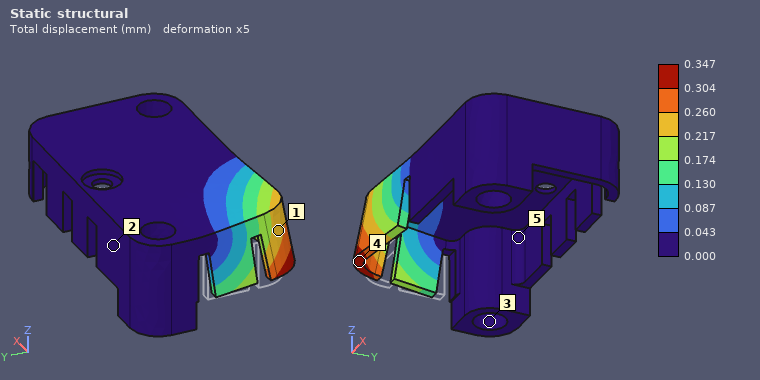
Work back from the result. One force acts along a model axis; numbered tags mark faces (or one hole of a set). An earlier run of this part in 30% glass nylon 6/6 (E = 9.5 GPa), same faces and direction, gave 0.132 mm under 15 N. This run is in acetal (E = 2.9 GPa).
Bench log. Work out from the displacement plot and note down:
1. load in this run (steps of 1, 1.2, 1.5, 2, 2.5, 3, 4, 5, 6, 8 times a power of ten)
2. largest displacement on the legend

12 N
0.347 mm
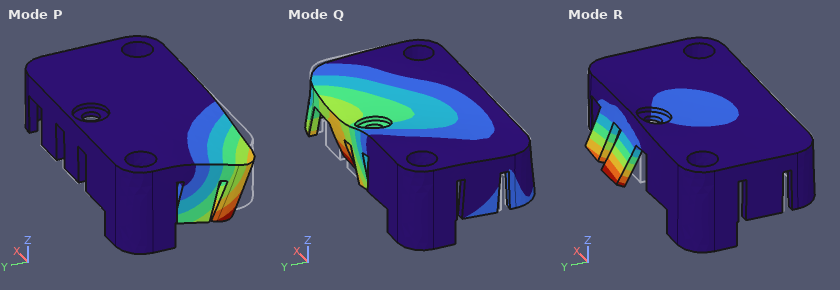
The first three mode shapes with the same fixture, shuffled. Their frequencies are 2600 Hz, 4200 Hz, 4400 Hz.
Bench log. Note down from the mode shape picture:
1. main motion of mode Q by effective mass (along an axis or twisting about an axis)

along Z
